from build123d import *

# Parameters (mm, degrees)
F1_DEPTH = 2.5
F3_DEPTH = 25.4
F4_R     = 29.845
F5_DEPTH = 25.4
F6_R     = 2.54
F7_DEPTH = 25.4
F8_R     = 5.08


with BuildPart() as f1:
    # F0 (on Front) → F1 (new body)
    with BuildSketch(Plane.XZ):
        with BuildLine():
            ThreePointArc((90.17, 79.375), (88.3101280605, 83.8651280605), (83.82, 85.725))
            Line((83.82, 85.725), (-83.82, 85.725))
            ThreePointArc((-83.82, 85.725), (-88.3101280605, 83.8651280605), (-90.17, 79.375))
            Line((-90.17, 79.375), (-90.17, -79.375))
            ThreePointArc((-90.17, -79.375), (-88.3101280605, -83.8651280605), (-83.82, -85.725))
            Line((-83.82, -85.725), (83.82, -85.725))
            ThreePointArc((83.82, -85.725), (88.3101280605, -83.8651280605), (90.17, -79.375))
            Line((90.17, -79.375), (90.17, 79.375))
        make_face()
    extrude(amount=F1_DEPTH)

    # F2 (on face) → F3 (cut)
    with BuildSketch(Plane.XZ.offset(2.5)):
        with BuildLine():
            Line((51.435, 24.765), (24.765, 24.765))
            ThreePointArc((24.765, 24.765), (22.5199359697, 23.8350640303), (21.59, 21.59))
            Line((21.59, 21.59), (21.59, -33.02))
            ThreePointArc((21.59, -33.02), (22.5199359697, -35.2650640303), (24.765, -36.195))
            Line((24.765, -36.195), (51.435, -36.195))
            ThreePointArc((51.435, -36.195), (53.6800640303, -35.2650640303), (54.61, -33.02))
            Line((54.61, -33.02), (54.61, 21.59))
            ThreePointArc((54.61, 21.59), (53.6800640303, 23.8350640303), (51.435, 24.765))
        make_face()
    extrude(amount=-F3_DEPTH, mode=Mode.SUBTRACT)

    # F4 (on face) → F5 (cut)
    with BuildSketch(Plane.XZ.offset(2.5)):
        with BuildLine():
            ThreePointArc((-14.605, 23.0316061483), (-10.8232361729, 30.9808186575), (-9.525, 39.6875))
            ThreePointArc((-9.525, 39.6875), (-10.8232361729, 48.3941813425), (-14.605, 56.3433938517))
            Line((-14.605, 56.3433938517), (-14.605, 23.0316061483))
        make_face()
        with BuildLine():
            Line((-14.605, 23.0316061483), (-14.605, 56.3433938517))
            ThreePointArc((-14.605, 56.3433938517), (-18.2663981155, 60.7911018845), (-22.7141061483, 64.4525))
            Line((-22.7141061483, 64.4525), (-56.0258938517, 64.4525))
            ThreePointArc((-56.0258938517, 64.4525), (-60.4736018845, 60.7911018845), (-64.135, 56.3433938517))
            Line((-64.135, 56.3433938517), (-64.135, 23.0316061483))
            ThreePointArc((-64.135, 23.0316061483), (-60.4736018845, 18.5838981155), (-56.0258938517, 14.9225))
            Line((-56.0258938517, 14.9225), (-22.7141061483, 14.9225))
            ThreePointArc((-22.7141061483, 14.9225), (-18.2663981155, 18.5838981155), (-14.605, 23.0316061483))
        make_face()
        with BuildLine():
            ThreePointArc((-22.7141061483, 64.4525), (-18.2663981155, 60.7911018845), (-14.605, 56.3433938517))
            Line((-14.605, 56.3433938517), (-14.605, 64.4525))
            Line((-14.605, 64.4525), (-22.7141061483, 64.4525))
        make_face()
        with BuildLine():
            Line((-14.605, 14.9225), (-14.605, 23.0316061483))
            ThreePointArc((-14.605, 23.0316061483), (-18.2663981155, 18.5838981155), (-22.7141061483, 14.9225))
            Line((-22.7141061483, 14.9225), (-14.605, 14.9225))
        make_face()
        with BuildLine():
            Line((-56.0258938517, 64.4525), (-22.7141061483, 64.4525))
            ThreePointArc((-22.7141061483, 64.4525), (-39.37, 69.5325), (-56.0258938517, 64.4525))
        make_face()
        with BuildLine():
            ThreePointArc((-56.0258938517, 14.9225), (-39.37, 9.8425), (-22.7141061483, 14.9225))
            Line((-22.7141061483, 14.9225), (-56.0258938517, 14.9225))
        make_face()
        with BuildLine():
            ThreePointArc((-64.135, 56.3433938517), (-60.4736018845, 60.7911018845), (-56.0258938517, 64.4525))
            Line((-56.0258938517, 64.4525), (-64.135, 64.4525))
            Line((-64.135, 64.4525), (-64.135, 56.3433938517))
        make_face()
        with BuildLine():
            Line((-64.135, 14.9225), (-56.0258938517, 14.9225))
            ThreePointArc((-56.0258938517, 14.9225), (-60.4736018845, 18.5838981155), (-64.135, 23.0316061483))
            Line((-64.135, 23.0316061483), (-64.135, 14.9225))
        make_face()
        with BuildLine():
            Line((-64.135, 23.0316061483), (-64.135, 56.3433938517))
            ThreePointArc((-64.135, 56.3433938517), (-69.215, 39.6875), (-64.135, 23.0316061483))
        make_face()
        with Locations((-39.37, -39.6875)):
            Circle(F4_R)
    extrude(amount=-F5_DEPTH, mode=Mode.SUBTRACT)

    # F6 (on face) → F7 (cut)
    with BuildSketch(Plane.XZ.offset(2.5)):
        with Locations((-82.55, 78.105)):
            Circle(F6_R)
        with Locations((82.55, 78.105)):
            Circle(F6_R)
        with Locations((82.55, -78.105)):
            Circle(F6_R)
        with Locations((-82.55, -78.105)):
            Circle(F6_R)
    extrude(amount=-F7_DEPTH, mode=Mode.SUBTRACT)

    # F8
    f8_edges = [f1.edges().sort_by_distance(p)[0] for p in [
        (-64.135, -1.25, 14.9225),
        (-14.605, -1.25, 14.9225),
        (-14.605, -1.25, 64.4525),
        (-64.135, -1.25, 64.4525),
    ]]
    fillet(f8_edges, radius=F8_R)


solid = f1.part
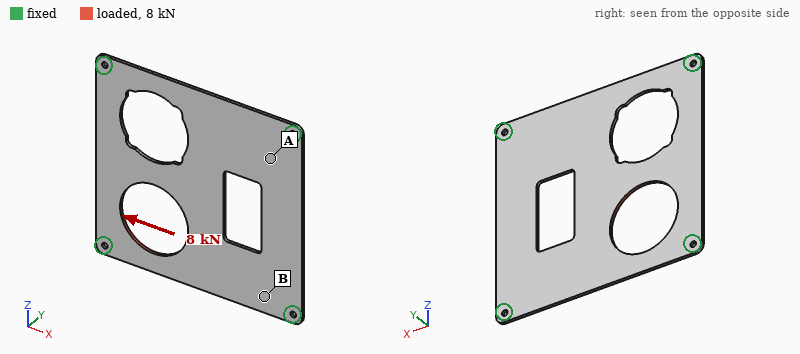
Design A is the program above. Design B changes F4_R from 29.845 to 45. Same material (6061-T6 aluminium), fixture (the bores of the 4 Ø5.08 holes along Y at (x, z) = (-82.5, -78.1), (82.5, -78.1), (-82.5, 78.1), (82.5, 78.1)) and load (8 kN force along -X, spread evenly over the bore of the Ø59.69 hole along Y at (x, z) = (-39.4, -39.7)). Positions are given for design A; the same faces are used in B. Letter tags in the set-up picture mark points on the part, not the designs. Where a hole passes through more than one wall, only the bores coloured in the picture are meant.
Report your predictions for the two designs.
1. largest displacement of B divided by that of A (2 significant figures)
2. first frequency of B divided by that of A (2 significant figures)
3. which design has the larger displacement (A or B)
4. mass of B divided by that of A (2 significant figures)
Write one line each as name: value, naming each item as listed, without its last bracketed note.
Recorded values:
largest displacement of B divided by that of A: 3.0
first frequency of B divided by that of A: 0.97
which design has the larger displacement: B
mass of B divided by that of A: 0.85
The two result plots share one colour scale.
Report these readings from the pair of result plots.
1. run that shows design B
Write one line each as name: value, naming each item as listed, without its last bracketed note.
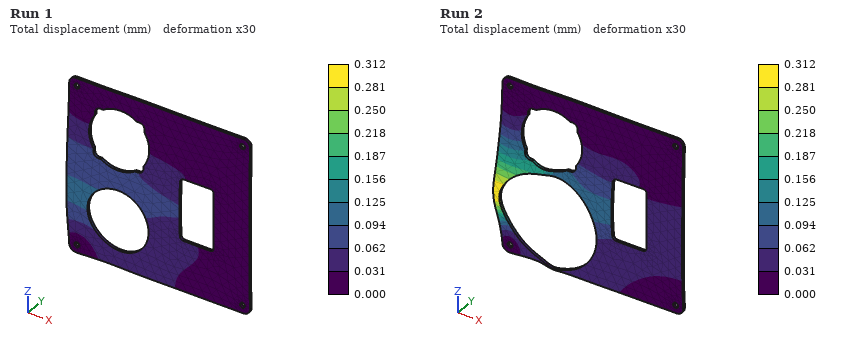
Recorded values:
run that shows design B: Run 2
